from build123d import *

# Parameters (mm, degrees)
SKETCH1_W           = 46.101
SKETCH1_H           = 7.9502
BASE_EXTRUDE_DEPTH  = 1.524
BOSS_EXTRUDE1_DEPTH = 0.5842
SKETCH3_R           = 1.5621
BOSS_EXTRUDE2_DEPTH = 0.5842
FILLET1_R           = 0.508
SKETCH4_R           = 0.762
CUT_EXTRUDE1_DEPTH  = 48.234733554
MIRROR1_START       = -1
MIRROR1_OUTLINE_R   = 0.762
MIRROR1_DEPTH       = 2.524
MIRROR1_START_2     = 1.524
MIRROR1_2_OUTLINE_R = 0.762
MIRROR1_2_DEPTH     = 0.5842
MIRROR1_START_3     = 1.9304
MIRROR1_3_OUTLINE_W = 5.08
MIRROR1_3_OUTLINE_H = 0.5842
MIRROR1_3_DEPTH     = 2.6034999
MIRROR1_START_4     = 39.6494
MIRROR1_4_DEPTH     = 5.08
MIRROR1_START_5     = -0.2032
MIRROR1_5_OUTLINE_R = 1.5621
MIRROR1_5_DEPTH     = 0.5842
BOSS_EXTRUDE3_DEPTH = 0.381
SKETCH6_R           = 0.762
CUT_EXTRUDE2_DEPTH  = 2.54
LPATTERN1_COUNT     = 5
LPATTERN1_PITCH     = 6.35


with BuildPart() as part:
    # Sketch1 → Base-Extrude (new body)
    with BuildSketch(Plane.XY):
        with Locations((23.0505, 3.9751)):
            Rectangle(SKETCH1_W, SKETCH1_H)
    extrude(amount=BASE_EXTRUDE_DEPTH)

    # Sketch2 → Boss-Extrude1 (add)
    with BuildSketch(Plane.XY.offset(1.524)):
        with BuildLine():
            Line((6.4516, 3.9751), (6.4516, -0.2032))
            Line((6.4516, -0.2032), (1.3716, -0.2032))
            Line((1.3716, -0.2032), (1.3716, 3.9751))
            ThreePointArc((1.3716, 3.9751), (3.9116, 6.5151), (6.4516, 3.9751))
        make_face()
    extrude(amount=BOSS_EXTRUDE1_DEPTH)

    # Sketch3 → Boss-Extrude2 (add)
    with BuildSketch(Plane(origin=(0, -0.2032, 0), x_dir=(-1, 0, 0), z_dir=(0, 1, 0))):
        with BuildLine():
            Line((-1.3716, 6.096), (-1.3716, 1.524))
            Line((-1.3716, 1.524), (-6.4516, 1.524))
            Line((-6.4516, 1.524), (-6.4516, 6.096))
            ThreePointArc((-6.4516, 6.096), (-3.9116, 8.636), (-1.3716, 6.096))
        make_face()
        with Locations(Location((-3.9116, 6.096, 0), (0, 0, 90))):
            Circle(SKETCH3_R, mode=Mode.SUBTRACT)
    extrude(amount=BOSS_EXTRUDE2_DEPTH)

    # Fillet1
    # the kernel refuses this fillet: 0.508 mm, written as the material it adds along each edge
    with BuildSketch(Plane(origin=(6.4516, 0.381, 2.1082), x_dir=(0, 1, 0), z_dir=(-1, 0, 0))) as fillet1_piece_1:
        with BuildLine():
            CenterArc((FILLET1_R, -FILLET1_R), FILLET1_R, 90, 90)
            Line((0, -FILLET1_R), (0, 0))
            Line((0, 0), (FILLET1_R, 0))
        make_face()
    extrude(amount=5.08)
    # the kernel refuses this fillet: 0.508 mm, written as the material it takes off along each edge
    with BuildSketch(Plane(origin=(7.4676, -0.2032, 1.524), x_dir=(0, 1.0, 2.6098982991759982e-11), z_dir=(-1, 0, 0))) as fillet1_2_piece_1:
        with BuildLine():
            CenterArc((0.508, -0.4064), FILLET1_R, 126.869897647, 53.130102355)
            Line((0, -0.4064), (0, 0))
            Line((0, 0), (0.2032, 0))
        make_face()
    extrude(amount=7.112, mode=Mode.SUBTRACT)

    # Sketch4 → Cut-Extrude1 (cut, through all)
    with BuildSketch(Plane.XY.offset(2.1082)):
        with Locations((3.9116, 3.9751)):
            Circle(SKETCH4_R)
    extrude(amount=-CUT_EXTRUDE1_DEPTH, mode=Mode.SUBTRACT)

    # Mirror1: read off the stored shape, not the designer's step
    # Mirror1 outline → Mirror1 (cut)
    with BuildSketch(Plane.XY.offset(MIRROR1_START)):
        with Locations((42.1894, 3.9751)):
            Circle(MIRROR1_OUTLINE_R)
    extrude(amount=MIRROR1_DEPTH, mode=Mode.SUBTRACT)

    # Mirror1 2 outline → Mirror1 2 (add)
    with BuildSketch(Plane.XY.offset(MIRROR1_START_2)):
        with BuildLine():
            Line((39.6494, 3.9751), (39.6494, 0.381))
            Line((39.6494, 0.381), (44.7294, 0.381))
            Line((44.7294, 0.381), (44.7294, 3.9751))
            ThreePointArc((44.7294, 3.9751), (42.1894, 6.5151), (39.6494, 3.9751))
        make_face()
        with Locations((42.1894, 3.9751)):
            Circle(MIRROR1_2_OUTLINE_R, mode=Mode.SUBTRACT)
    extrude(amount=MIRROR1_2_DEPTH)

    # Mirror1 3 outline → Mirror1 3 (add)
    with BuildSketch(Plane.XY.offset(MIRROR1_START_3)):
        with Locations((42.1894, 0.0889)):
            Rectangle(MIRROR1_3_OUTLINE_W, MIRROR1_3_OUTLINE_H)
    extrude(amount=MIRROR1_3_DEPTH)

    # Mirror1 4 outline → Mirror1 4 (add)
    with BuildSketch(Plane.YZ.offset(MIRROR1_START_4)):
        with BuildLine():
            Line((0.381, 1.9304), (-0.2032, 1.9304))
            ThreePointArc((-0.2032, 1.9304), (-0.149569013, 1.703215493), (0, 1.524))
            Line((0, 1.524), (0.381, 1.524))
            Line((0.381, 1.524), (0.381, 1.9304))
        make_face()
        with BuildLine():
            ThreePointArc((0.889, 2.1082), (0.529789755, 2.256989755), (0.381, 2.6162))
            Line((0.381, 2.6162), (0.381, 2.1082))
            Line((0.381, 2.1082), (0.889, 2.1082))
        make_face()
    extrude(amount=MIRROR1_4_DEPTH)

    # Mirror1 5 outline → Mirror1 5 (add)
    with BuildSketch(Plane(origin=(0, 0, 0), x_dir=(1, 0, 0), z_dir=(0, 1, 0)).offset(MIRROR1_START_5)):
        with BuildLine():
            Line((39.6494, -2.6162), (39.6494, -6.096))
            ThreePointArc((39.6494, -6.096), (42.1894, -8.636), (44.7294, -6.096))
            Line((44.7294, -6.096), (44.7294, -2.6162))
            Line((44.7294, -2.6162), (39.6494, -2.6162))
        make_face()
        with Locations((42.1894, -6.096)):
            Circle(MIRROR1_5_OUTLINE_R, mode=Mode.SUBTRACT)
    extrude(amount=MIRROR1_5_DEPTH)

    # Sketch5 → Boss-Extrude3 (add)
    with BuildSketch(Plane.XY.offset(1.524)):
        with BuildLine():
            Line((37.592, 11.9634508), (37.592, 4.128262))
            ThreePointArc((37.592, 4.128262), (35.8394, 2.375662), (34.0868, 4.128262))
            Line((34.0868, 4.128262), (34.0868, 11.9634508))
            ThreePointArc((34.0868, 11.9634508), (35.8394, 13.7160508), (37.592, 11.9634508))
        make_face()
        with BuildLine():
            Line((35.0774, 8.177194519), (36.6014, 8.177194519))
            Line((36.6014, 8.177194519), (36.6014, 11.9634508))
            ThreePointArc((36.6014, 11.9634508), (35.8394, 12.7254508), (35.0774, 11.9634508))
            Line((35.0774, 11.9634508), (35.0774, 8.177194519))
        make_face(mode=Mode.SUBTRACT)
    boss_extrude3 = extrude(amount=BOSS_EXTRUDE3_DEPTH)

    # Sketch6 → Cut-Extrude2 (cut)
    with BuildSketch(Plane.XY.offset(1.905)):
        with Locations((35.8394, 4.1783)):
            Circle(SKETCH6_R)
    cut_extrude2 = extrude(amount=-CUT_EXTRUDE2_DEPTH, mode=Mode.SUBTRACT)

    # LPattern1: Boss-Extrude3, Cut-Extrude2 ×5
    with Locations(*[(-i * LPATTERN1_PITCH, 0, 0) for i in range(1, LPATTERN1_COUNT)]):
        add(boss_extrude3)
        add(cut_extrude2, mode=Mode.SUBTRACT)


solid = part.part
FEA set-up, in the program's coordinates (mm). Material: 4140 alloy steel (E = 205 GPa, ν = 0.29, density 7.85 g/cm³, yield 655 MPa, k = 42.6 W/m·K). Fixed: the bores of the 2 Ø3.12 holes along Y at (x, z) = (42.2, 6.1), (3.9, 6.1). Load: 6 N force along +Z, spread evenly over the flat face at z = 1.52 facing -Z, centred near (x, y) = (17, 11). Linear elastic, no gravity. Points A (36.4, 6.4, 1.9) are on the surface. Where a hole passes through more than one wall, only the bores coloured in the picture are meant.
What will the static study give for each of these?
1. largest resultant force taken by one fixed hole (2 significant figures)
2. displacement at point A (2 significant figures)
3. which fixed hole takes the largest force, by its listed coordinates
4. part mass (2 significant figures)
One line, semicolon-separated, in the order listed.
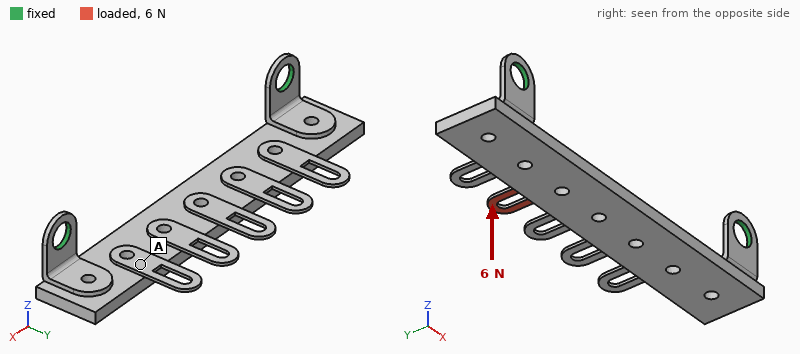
5.5 N; 0.032 mm; (3.9, 6.1); 5.1 g
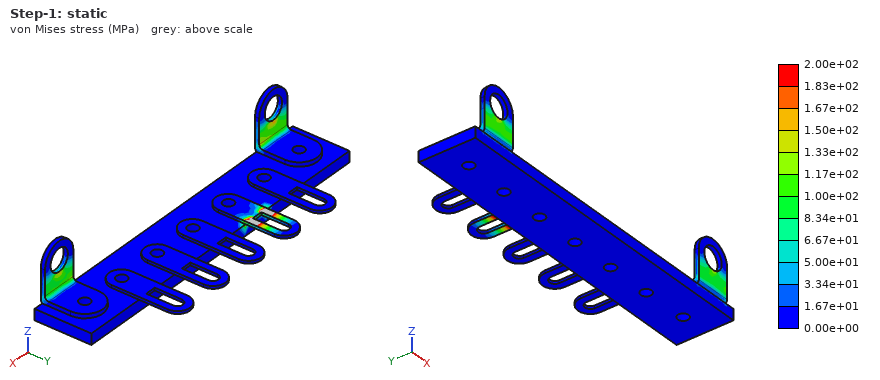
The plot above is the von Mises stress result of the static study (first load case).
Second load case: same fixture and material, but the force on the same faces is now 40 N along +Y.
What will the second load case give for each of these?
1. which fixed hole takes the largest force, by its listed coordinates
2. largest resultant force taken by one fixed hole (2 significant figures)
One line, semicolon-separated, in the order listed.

(3.9, 6.1); 29 N
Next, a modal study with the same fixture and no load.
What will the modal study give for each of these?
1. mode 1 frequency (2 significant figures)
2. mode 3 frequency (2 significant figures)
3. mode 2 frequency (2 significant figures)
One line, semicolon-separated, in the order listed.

1500 Hz; 6000 Hz; 5400 Hz
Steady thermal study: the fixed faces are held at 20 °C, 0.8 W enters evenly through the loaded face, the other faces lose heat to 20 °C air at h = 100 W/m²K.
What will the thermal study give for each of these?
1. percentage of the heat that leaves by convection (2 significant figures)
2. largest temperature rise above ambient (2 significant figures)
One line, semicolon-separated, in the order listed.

78 %; 76 K
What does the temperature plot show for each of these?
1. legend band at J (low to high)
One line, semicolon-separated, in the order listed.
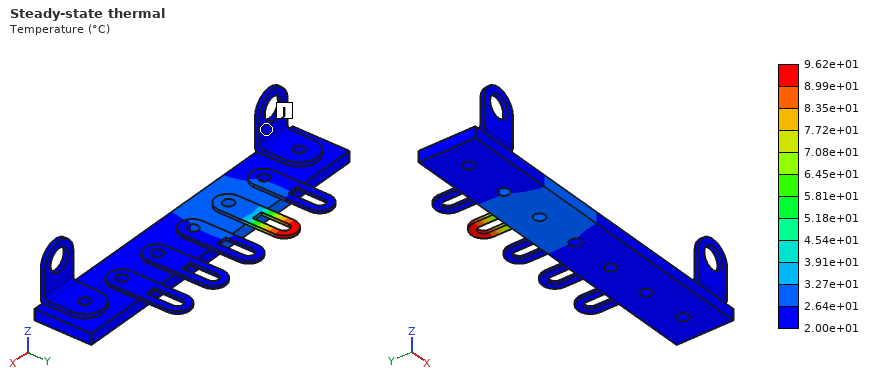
2.00e+01 to 2.64e+01 °C
